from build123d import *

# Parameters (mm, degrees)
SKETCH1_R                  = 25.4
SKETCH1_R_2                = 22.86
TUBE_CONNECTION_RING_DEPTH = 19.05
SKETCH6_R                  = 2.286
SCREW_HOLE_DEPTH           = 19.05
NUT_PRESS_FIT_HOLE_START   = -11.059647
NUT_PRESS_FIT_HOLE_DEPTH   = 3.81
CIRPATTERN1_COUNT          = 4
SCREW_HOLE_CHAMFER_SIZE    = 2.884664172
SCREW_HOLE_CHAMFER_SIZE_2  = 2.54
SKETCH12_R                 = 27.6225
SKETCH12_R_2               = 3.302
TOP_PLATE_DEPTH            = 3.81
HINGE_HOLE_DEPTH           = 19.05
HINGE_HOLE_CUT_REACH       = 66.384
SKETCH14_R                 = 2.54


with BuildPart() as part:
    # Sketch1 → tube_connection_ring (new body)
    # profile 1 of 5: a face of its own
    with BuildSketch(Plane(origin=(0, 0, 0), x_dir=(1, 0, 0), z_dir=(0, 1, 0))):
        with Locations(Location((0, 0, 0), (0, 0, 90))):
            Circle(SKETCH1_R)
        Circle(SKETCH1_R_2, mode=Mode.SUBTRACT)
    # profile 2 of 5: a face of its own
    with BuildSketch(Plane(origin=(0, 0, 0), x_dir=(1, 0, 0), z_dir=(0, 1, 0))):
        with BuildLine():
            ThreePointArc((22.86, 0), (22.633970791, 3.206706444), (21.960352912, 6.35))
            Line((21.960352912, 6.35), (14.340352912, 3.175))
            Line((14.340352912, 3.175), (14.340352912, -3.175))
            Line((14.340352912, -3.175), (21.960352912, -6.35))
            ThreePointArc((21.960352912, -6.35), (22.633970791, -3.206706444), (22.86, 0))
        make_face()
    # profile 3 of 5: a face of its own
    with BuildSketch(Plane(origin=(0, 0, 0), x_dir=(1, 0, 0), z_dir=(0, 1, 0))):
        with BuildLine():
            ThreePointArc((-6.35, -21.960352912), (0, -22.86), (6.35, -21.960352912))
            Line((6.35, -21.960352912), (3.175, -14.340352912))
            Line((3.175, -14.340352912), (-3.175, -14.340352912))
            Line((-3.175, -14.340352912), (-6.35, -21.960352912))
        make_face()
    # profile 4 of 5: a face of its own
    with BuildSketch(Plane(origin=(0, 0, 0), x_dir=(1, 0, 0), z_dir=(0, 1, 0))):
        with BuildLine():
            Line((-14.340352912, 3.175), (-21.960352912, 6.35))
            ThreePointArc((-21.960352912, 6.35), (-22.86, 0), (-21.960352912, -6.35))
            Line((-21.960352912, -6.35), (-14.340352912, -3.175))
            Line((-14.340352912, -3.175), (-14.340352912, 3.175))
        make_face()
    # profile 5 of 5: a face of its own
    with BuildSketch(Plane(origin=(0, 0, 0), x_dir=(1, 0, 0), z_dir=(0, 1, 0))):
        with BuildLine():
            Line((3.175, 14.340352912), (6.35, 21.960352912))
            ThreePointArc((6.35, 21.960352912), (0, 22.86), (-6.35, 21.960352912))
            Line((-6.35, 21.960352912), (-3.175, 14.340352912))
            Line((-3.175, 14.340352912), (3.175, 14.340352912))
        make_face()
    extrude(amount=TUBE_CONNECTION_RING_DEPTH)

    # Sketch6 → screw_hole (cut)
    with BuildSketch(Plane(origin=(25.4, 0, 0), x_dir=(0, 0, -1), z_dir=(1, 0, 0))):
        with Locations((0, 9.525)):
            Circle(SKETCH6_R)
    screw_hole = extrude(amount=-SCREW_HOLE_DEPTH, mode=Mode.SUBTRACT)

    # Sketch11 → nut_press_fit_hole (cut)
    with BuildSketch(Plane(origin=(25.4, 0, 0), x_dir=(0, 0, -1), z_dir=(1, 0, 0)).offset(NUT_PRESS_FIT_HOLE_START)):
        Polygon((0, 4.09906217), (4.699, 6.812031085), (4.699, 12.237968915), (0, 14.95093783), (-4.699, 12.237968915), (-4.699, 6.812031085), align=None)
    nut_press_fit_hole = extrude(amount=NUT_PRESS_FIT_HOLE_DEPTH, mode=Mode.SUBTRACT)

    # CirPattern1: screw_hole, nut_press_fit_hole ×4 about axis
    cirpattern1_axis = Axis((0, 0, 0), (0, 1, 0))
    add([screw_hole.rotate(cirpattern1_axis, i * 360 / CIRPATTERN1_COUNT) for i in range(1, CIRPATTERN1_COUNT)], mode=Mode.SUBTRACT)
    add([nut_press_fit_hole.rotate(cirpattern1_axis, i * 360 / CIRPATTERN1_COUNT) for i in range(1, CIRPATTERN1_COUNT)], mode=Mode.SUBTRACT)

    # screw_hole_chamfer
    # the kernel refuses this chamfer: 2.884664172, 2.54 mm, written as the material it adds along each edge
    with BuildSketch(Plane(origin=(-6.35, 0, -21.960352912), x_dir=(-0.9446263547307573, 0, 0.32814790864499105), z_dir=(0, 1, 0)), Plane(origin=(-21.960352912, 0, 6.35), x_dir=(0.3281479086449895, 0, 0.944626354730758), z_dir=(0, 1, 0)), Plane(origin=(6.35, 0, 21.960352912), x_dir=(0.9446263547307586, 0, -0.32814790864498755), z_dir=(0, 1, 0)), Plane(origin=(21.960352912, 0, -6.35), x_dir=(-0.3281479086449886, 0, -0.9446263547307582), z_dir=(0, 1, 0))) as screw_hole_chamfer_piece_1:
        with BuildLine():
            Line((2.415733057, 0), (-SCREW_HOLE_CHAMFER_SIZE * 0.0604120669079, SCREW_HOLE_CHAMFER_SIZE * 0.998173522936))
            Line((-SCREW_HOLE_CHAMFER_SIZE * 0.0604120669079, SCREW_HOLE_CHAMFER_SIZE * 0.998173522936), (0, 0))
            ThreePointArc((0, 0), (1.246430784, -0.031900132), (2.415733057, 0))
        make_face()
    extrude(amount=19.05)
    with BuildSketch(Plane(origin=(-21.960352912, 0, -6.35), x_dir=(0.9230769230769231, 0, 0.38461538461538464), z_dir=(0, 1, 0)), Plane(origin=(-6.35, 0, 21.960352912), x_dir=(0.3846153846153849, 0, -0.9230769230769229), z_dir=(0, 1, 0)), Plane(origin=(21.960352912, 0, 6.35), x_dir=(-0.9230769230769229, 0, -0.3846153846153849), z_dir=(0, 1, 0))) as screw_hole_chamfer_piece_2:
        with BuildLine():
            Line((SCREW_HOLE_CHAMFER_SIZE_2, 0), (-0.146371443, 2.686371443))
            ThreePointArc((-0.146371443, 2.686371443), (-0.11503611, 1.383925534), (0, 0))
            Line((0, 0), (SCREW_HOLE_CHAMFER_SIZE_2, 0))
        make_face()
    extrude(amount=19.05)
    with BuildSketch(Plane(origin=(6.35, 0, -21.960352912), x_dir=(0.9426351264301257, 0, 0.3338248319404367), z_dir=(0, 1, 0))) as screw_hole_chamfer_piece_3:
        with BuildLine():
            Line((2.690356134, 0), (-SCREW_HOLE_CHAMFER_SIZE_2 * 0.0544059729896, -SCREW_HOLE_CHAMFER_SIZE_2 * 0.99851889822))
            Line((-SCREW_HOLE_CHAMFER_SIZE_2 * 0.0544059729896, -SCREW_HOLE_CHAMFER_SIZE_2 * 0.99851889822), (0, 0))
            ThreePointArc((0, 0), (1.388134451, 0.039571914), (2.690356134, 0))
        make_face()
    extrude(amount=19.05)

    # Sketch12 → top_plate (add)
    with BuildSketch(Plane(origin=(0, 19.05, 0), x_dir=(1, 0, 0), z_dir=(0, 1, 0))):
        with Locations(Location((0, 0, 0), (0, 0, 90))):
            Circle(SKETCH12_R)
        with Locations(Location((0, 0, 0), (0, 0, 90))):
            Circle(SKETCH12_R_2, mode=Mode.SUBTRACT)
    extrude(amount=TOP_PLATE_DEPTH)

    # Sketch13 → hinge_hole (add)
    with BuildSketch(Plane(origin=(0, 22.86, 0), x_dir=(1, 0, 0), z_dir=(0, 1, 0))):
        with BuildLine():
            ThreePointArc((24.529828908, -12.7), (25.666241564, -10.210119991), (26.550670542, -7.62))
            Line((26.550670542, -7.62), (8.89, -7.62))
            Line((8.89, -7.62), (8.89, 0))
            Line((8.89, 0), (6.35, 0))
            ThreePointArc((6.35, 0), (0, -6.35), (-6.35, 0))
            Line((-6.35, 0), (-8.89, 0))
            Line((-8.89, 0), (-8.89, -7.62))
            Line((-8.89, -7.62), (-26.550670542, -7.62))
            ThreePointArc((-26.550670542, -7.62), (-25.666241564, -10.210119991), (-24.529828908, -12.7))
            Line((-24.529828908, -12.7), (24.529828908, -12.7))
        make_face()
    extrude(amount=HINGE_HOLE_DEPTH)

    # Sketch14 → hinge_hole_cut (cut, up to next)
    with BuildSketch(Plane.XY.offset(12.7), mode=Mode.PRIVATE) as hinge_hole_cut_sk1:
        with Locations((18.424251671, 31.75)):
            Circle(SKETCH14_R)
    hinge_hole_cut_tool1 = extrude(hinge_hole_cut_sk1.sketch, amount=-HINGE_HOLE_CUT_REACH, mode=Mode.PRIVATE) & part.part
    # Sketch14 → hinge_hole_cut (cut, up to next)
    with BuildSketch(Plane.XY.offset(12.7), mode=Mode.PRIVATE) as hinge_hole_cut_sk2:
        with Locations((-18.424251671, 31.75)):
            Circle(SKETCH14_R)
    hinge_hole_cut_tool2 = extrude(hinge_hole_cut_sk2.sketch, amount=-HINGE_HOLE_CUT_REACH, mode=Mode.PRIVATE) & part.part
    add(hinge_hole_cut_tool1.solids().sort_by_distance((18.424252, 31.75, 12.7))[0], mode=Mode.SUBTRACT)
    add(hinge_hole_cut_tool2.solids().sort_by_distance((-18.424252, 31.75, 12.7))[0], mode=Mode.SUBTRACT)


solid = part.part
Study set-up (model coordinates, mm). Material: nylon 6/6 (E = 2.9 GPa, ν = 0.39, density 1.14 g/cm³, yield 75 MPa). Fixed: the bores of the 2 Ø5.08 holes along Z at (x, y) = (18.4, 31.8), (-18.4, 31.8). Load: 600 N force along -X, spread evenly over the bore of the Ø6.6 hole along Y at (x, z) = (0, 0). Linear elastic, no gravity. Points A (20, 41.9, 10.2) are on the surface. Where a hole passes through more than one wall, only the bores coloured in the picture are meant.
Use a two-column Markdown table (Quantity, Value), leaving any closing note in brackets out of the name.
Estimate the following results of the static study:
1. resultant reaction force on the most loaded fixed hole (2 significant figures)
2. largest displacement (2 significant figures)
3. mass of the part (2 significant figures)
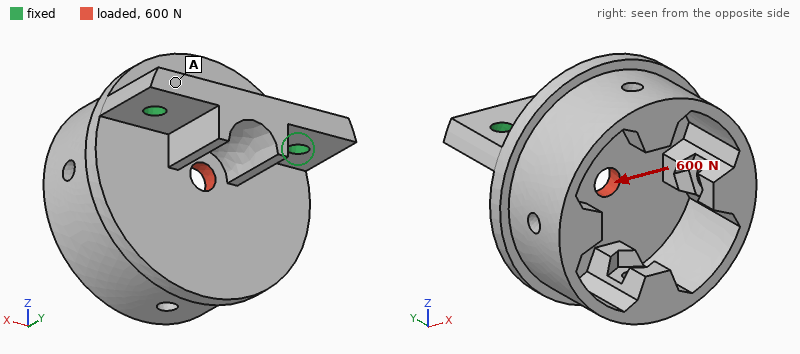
| Quantity | Value |
|---|---|
| resultant reaction force on the most loaded fixed hole | 380 N |
| largest displacement | 0.14 mm |
| mass of the part | 31 g |
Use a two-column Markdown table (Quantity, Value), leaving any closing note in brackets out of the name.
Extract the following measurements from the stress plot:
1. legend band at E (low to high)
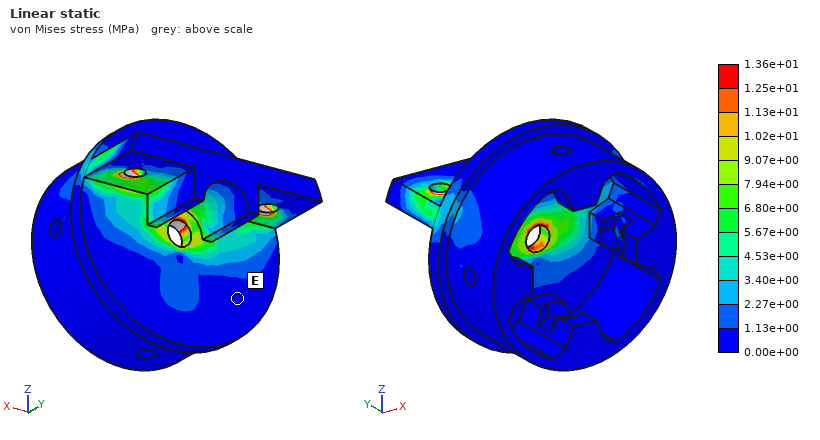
| Quantity | Value |
|---|---|
| legend band at E | 0.00e+00 to 1.13e+00 MPa |
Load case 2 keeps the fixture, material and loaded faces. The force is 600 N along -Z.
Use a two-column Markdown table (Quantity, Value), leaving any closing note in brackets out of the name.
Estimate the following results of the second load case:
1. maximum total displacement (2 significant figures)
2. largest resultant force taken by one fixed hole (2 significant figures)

| Quantity | Value |
|---|---|
| maximum total displacement | 0.80 mm |
| largest resultant force taken by one fixed hole | 300 N |
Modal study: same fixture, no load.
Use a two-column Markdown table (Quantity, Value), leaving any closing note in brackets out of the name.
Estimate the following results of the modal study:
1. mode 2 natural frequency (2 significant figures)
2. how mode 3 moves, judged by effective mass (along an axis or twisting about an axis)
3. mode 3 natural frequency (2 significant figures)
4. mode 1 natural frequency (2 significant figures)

| Quantity | Value |
|---|---|
| mode 2 natural frequency | 1800 Hz |
| how mode 3 moves, judged by effective mass | along X |
| mode 3 natural frequency | 1900 Hz |
| mode 1 natural frequency | 600 Hz |
